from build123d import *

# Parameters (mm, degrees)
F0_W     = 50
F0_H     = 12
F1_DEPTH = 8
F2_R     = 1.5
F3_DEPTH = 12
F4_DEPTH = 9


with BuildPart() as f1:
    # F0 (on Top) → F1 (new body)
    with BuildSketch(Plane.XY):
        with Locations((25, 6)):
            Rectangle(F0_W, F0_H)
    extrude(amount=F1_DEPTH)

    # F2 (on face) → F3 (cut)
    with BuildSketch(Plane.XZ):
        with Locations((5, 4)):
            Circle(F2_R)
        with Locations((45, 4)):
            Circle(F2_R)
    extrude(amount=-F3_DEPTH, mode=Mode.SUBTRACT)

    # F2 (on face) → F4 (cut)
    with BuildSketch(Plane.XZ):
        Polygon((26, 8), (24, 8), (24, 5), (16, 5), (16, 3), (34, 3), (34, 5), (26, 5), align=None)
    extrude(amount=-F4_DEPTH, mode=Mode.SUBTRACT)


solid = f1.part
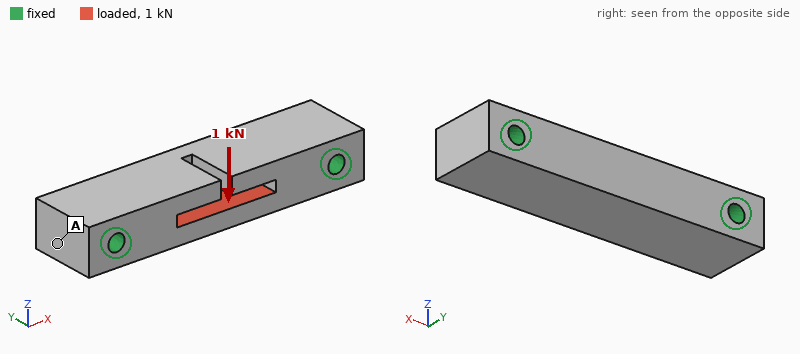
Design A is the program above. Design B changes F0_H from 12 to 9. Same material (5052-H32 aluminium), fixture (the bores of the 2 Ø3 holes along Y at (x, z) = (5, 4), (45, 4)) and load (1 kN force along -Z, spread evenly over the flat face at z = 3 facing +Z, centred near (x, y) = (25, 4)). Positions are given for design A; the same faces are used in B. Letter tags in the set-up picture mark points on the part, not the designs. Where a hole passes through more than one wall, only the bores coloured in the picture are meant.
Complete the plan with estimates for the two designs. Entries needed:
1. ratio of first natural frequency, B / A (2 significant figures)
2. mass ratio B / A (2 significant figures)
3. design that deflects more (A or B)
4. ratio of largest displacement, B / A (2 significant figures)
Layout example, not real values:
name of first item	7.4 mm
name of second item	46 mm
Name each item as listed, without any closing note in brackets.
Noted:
ratio of first natural frequency, B / A	0.99
mass ratio B / A	0.74
design that deflects more	B
ratio of largest displacement, B / A	1.2
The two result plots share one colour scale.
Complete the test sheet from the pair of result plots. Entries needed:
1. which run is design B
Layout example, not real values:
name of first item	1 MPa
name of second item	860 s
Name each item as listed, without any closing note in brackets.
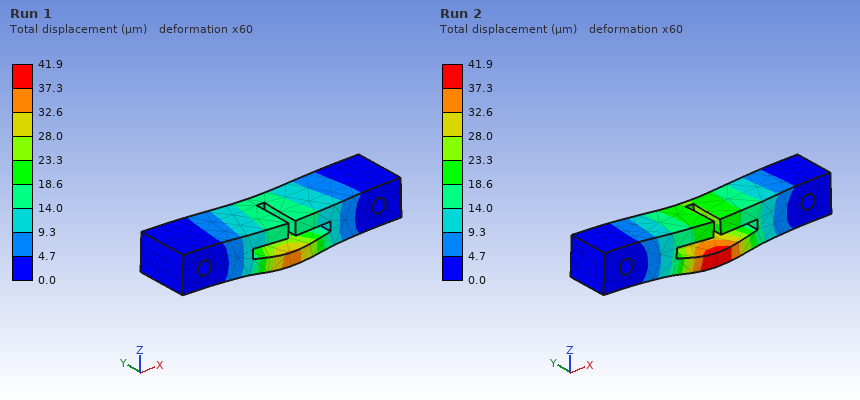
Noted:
which run is design B	Run 2
